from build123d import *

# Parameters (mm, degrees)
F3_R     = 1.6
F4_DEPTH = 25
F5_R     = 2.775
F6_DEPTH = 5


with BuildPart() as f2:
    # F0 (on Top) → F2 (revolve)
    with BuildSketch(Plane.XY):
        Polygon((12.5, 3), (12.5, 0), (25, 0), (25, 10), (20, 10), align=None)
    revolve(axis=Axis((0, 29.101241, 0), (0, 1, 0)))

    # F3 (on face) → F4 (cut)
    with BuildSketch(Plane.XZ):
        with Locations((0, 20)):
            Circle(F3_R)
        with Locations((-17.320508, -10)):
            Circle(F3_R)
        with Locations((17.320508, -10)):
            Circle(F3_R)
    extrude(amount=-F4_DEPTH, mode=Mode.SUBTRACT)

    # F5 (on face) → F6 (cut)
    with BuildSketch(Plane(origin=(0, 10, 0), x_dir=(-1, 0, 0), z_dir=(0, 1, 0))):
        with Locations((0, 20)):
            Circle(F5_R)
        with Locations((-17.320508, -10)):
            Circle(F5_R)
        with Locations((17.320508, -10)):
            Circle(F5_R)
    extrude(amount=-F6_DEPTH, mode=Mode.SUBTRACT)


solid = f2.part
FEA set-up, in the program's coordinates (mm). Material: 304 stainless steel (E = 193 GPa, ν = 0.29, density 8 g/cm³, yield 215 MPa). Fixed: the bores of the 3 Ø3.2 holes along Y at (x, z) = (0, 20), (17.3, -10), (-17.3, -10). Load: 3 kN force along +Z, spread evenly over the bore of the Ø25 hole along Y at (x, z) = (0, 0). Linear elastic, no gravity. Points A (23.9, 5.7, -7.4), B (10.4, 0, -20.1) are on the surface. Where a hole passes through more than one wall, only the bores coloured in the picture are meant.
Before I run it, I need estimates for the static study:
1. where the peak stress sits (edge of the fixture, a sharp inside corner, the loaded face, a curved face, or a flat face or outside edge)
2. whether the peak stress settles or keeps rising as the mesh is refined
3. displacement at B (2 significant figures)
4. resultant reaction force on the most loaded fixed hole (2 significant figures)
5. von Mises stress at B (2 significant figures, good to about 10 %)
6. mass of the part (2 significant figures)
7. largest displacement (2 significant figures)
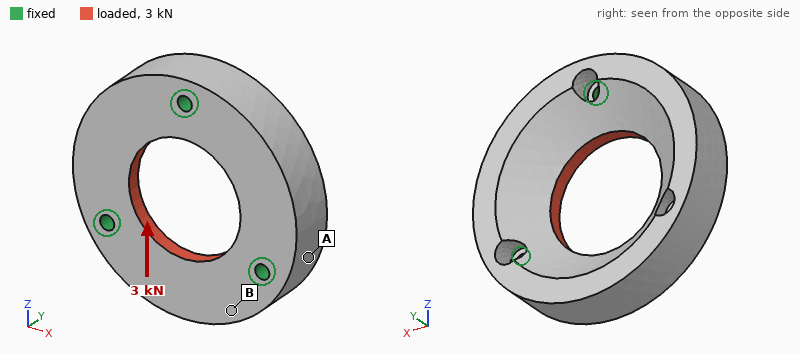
edge of the fixture
keeps rising
1.3 µm
1.1 kN
9.9 MPa
94 g
2.4 µm
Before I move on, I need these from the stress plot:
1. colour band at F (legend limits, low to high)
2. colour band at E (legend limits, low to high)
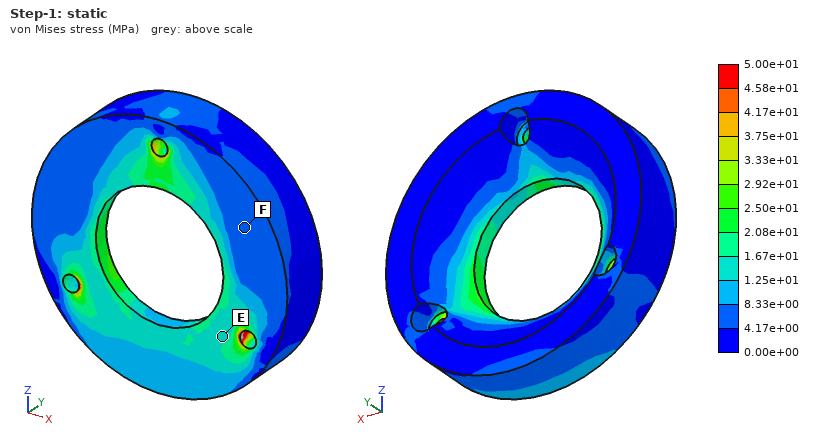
4.17e+00 to 8.33e+00 MPa
1.25e+01 to 1.67e+01 MPa
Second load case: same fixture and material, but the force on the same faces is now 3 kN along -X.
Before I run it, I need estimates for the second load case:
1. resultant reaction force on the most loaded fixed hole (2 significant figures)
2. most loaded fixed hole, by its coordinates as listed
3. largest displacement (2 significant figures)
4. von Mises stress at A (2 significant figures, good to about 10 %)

1.2 kN
(0, 20)
2.1 µm
6.2 MPa
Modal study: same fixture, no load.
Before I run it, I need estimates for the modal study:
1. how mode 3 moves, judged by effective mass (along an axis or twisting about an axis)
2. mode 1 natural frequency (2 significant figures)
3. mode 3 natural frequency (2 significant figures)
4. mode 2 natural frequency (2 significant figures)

along Y
11 kHz
15 kHz
11 kHz
